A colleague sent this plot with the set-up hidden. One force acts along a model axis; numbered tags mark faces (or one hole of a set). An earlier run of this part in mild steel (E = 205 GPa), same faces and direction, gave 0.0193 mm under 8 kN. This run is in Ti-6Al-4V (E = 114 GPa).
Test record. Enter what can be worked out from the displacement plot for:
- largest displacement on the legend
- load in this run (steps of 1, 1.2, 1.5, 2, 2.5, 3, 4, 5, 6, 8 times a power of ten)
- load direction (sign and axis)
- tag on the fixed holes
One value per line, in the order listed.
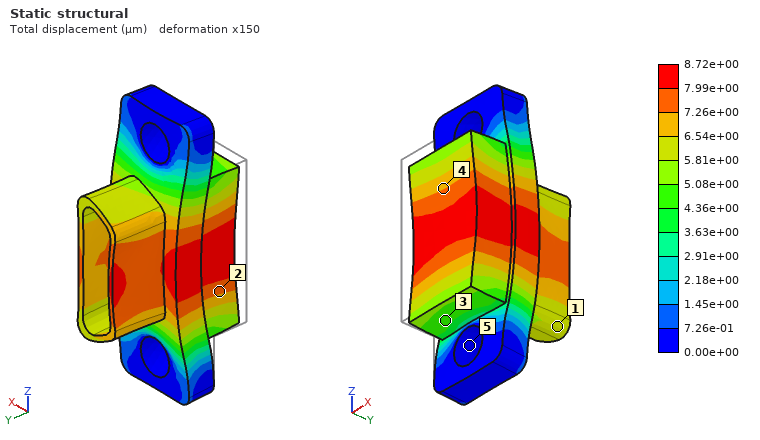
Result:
8.72e+00 µm
2 kN
+Y
5
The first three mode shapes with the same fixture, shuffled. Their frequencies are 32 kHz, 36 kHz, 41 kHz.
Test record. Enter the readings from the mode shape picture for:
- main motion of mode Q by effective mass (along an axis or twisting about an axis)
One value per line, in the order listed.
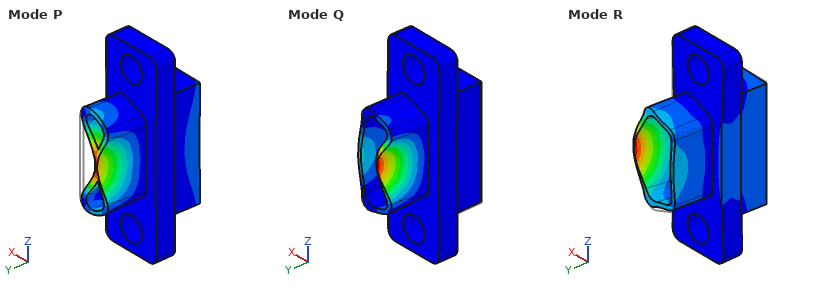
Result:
along X
